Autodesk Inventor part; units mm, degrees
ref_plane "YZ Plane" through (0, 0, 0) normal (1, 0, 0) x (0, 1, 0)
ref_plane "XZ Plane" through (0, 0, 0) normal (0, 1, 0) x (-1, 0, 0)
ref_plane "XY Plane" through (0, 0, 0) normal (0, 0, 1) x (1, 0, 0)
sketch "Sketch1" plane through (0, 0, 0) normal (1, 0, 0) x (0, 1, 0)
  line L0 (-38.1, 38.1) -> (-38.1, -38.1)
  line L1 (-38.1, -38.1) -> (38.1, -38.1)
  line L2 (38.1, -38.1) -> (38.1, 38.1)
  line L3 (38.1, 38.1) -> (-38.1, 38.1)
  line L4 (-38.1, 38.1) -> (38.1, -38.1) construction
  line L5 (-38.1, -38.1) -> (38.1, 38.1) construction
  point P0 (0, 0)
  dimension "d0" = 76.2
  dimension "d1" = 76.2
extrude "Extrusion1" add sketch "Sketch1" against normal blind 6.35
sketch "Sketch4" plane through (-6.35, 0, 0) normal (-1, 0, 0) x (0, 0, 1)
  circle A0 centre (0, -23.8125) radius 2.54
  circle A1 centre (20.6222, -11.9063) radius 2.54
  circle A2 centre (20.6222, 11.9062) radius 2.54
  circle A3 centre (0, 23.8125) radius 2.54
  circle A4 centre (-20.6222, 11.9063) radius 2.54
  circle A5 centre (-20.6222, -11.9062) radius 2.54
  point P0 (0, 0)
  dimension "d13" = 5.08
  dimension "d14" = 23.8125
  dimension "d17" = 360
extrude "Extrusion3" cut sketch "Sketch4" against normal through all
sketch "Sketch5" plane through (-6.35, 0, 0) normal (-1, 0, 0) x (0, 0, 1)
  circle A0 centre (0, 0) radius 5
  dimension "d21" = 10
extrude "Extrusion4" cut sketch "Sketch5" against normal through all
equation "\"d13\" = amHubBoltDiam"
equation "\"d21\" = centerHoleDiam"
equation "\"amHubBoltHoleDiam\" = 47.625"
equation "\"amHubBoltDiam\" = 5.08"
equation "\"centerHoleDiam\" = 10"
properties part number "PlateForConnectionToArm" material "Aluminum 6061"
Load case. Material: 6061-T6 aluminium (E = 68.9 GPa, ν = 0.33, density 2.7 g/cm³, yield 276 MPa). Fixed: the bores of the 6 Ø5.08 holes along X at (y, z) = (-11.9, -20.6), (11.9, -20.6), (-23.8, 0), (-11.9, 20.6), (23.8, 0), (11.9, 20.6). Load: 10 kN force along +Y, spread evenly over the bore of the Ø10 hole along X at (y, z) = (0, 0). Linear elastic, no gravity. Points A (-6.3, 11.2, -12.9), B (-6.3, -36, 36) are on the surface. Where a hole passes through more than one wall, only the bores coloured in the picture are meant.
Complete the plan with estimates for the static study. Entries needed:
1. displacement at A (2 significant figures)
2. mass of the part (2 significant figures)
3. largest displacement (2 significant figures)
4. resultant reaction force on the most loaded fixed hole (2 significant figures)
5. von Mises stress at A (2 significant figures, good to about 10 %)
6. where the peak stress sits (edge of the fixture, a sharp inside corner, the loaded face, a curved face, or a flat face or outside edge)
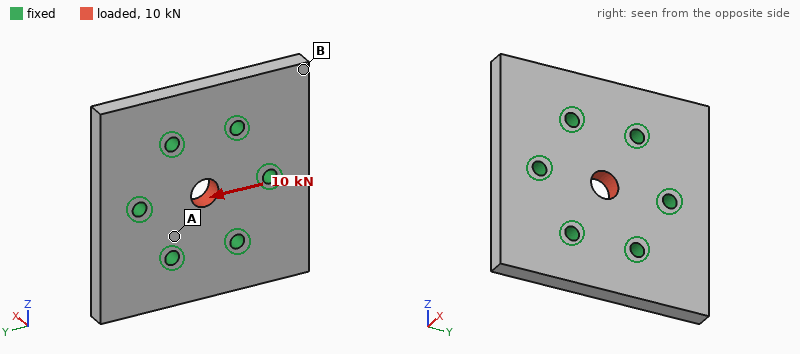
2.5 µm
96 g
9.8 µm
2.6 kN
16 MPa
the loaded face
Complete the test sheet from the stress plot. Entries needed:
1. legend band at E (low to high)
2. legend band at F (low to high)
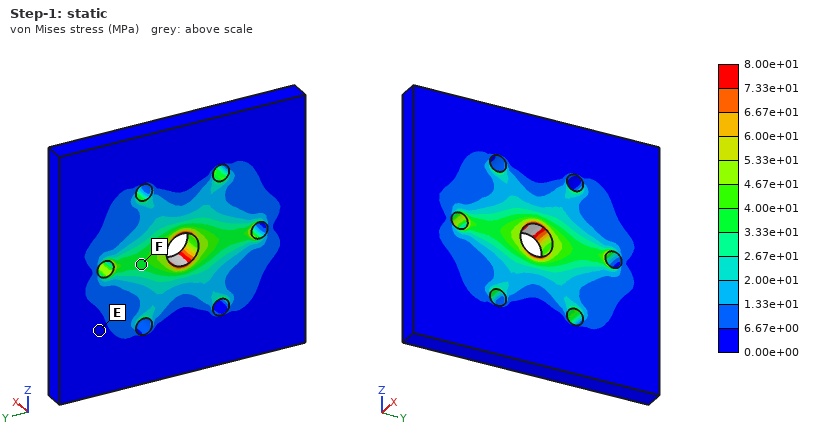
0.00e+00 to 6.67e+00 MPa
3.33e+01 to 4.00e+01 MPa
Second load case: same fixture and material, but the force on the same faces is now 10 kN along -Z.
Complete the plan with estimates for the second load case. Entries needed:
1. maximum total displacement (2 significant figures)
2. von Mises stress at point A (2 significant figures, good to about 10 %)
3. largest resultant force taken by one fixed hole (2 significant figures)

9.9 µm
25 MPa
2.3 kN
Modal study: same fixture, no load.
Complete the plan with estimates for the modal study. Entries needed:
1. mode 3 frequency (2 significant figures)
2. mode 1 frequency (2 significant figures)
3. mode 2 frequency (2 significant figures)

8600 Hz
8300 Hz
8400 Hz
